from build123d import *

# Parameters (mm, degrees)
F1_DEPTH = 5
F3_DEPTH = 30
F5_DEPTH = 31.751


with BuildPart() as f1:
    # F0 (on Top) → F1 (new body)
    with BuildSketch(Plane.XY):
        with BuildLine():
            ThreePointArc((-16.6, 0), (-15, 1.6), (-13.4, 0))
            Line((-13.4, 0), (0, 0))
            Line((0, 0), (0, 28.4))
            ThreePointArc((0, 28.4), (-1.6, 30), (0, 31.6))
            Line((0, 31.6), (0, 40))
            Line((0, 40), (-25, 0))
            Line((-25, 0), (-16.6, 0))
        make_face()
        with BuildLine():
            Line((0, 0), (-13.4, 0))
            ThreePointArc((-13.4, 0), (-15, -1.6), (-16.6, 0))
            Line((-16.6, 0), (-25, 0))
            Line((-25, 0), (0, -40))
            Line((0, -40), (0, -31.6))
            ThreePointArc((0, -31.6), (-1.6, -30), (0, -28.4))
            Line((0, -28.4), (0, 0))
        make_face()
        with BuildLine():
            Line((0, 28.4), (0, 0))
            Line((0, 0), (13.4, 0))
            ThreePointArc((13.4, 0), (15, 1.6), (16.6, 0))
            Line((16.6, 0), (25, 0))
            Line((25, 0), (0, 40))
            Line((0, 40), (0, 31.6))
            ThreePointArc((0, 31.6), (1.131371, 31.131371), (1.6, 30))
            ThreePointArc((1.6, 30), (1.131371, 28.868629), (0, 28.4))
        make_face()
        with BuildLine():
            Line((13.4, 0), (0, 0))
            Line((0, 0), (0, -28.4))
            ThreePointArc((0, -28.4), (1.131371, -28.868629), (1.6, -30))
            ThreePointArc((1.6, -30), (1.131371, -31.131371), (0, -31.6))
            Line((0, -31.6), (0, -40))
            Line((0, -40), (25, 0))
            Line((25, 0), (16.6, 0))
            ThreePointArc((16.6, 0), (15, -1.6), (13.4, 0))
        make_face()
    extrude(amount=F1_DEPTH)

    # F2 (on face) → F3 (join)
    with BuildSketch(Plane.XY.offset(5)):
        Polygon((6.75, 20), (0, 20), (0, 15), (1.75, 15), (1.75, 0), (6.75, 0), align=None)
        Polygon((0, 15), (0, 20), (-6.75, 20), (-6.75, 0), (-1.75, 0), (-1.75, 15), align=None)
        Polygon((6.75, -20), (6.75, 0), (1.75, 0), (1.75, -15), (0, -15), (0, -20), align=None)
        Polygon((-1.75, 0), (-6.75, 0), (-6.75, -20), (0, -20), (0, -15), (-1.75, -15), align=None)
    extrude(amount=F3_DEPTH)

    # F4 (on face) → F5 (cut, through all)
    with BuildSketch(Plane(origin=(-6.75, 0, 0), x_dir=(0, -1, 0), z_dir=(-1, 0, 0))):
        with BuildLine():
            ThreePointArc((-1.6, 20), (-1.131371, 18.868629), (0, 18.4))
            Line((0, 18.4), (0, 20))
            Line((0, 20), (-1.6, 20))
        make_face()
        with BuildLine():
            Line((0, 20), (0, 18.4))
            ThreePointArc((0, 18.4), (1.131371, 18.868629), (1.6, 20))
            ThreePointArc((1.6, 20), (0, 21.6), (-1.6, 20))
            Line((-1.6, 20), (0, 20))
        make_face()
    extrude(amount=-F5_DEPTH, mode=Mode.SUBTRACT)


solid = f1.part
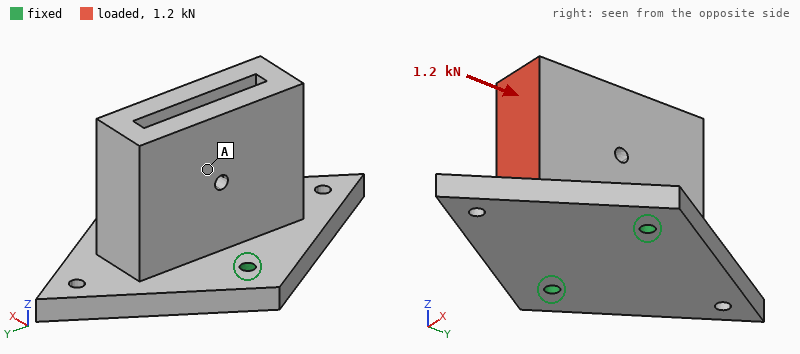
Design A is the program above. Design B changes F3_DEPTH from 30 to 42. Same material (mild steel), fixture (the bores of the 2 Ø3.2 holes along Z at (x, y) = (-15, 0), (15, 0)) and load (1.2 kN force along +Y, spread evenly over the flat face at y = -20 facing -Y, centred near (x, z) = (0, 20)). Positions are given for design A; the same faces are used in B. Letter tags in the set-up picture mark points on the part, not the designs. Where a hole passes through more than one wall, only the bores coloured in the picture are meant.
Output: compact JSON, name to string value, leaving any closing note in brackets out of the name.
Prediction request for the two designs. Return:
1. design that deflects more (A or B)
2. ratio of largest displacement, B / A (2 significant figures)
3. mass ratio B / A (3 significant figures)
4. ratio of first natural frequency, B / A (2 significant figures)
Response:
{"design that deflects more": "B", "ratio of largest displacement, B / A": "1.6", "mass ratio B / A": "1.23", "ratio of first natural frequency, B / A": "0.72"}
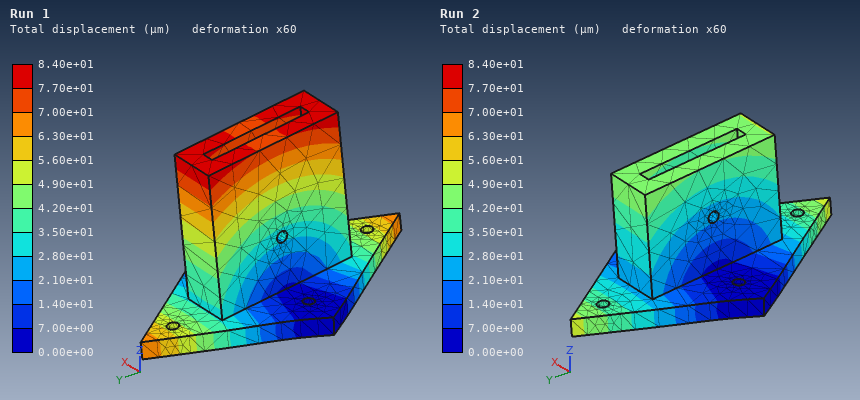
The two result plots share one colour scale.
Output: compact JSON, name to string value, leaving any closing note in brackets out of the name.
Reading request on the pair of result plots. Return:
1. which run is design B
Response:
{"which run is design B": "Run 1"}
